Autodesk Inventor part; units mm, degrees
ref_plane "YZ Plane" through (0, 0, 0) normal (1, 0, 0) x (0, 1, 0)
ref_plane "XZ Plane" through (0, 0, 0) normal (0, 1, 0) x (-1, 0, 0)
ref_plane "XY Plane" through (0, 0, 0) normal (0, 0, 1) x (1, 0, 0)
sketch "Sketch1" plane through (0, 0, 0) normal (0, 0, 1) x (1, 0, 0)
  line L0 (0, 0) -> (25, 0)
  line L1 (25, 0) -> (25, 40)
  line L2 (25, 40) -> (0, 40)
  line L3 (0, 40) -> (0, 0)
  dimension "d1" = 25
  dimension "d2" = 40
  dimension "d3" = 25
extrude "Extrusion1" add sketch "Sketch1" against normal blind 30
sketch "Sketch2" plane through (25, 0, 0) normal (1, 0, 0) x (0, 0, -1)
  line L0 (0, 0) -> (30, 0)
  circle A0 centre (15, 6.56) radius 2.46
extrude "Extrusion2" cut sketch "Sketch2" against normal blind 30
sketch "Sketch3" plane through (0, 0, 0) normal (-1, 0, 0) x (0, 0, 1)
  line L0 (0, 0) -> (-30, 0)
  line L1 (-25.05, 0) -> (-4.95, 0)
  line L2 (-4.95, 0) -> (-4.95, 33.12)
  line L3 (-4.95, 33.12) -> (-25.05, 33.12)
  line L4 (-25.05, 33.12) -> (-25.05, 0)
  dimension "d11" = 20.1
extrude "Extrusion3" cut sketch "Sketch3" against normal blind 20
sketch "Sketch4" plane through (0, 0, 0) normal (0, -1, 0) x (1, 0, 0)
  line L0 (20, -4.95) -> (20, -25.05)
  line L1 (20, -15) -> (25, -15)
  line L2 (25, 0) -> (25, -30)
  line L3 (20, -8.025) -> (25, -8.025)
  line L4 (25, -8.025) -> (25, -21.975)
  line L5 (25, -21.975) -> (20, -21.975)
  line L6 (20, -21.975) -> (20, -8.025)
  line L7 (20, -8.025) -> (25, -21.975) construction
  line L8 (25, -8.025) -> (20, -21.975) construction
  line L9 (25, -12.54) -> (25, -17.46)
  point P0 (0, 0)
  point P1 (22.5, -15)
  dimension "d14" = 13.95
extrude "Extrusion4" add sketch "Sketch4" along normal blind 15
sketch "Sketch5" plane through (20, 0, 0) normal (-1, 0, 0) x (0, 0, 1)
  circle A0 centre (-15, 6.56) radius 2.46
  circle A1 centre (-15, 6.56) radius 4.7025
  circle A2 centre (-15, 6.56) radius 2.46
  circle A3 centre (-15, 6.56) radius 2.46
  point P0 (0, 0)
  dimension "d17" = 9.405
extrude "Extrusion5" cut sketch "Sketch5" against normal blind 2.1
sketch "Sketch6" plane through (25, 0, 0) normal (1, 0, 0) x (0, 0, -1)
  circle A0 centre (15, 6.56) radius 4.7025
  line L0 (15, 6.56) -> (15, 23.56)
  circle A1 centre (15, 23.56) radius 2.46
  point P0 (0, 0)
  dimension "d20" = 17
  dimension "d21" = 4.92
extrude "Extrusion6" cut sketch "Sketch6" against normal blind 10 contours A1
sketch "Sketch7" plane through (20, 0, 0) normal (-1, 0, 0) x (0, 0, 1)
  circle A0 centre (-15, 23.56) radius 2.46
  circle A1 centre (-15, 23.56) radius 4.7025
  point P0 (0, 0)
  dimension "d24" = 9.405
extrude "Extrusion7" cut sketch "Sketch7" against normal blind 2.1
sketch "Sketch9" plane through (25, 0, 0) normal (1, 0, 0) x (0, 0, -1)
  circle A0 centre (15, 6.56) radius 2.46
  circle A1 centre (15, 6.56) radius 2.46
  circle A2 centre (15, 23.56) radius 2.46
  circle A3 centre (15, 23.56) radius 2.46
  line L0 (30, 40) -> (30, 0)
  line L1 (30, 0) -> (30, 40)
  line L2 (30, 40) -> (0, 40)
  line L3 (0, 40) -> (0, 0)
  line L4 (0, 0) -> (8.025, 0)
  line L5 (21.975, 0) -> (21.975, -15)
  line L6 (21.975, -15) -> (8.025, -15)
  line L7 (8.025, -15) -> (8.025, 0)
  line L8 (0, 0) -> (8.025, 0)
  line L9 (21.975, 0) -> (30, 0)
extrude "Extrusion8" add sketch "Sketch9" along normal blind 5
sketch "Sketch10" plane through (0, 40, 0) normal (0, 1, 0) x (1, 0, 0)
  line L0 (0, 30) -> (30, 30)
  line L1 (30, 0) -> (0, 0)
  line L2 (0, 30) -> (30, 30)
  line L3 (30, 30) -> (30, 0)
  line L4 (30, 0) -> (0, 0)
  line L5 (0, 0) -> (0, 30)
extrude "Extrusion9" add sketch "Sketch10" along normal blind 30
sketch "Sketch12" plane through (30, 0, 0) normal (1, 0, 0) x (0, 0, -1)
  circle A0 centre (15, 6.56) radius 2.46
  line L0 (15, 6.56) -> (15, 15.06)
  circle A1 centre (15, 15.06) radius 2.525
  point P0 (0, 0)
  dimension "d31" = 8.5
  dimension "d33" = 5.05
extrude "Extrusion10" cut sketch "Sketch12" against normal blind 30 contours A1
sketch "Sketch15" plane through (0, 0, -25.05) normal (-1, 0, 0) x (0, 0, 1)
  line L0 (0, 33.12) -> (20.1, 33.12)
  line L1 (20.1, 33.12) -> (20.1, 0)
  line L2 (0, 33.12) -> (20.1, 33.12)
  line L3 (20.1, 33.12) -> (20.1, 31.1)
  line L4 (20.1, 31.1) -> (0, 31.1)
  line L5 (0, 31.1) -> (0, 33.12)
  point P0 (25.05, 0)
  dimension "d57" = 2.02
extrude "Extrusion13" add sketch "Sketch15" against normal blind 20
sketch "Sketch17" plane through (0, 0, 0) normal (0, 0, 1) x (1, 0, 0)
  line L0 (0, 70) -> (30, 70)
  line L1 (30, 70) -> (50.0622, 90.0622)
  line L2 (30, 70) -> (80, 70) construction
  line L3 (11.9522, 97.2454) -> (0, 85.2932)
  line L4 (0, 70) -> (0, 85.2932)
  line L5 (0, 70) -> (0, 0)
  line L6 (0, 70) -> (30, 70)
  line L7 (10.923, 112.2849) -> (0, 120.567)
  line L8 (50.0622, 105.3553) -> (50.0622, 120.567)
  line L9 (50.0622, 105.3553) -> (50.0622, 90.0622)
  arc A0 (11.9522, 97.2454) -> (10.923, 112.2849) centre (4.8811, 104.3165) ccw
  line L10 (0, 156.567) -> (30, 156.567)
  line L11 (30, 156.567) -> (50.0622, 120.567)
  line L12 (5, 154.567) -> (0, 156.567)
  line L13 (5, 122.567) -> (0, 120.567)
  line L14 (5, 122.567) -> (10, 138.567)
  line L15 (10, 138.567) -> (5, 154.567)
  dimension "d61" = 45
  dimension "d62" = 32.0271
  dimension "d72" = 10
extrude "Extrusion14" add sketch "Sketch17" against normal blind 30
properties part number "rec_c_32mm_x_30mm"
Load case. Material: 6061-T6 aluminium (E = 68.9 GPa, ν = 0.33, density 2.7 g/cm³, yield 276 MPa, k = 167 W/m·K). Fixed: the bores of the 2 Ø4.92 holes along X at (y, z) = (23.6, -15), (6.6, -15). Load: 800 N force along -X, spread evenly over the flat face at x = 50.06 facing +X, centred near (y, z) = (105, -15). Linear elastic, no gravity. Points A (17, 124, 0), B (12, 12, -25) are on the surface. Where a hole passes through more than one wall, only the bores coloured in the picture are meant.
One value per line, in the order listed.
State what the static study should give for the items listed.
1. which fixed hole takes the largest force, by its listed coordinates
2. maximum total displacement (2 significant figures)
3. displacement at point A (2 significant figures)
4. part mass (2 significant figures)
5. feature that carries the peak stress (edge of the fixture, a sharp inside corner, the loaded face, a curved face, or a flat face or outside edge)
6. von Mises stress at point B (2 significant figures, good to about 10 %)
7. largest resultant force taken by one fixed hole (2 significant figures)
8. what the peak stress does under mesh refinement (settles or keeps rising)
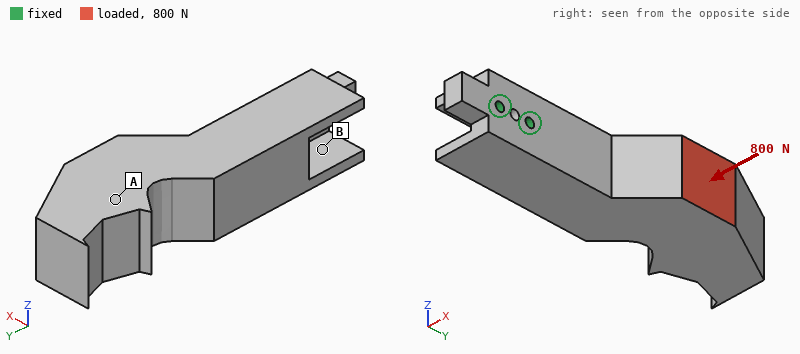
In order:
(23.6, -15)
0.25 mm
0.18 mm
400 g
edge of the fixture
21 MPa
3.4 kN
keeps rising
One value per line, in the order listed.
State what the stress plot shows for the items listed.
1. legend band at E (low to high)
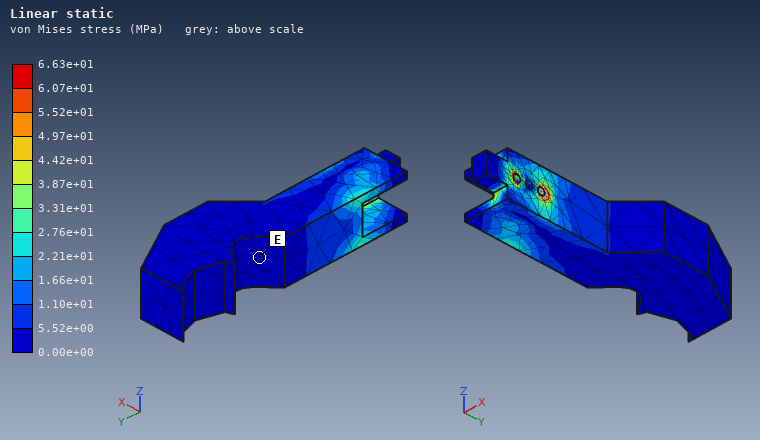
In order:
0.00e+00 to 5.52e+00 MPa
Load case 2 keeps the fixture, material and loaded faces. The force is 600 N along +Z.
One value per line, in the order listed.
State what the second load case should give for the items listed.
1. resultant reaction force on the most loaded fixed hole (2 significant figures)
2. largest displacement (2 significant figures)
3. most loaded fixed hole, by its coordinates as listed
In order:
2.7 kN
0.16 mm
(23.6, -15)
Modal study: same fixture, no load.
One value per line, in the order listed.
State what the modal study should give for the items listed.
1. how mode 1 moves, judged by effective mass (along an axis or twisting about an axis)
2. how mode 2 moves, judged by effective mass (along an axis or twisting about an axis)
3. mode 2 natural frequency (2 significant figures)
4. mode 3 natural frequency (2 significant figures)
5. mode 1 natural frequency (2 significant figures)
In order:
along X
along Z
730 Hz
2300 Hz
630 Hz
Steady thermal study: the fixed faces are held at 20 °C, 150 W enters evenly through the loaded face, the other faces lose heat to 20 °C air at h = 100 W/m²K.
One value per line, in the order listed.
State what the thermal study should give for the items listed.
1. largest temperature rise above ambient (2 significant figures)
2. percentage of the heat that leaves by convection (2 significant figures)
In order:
69 K
55 %
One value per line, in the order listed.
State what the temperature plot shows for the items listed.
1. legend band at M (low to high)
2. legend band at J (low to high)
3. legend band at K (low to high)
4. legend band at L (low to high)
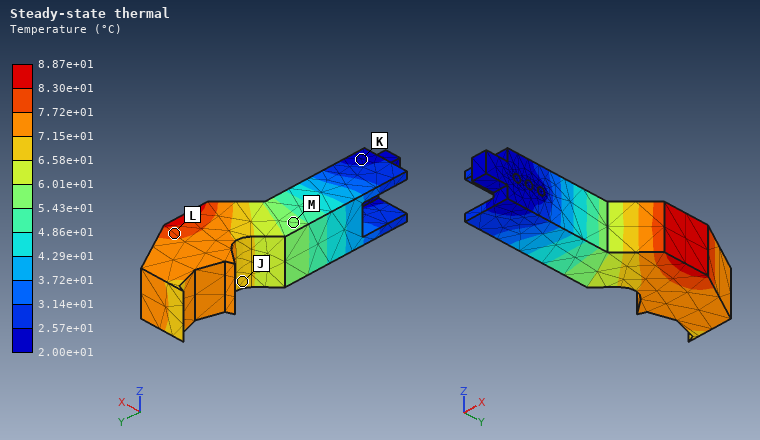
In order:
5.43e+01 to 6.01e+01 °C
6.58e+01 to 7.15e+01 °C
2.00e+01 to 2.57e+01 °C
7.72e+01 to 8.30e+01 °C
